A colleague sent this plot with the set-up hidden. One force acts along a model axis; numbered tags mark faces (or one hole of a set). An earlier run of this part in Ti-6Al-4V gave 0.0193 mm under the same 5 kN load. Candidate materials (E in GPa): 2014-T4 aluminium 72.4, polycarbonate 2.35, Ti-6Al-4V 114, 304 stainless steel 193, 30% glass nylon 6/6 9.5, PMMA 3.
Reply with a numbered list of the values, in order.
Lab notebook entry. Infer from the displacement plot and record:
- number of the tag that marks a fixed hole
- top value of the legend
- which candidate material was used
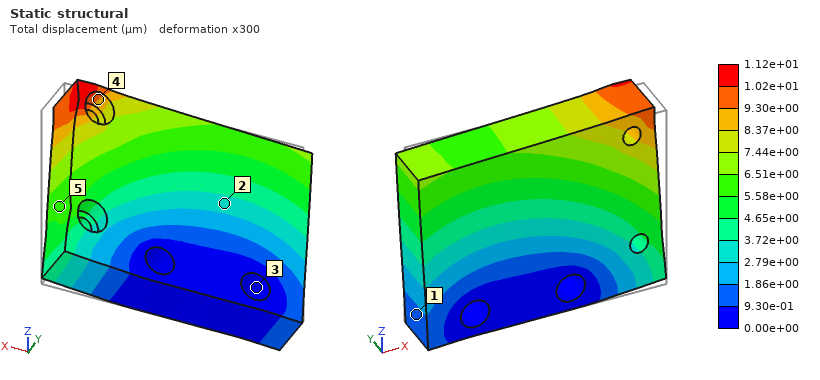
1. 3
2. 1.12e+01 µm
3. 304 stainless steel
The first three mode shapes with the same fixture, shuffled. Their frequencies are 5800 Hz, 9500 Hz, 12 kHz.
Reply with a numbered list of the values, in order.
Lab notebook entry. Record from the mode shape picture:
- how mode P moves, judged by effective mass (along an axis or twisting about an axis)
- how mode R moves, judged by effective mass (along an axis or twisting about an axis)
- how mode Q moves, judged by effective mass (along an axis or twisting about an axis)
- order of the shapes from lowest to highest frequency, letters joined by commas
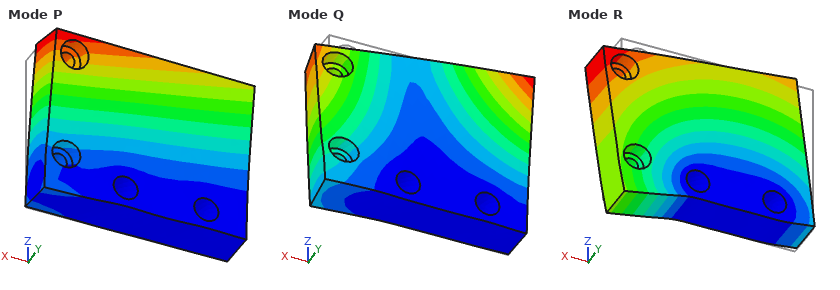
1. along Y
2. along X
3. twisting about Z
4. P, Q, R
